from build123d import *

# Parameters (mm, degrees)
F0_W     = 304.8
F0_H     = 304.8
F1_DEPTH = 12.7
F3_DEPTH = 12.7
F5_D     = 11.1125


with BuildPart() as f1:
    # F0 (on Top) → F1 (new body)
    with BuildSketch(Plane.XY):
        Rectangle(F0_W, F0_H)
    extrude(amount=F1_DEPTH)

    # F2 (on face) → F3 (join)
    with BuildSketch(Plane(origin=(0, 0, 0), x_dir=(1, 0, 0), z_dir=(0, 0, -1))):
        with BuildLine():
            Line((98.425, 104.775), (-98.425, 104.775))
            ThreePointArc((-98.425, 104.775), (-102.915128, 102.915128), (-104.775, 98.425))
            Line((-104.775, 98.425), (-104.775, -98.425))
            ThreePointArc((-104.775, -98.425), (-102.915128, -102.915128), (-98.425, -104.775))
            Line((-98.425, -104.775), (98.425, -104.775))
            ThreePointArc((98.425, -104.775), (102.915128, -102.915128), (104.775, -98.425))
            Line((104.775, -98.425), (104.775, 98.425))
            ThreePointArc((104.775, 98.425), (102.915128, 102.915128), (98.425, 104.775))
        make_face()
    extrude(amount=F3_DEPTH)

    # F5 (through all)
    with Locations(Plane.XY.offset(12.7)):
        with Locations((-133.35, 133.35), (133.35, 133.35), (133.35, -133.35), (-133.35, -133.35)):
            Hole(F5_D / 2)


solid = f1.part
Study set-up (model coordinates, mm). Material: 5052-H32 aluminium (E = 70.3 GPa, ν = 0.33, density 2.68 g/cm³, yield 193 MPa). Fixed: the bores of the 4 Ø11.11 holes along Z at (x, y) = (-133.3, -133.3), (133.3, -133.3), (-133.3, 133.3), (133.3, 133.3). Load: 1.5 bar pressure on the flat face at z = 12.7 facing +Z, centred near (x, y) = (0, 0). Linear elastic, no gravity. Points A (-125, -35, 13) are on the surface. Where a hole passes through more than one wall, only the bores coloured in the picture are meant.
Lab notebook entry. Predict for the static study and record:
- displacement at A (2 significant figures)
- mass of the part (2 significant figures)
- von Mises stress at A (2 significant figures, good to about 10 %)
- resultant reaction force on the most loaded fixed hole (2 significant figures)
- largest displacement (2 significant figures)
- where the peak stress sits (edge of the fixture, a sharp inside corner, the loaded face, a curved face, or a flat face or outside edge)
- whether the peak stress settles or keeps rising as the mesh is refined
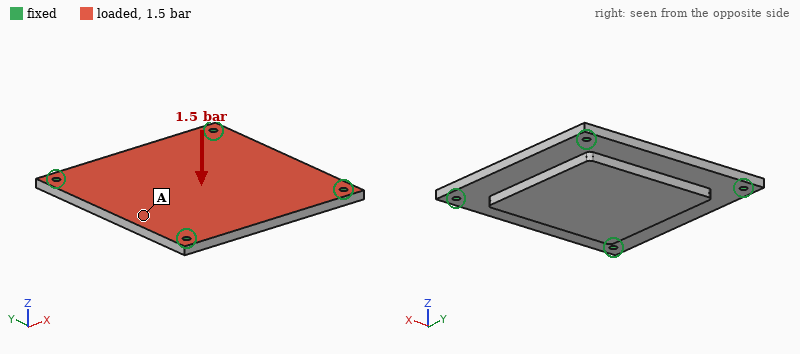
0.12 mm
4.6 kg
10 MPa
4.6 kN
0.16 mm
edge of the fixture
keeps rising
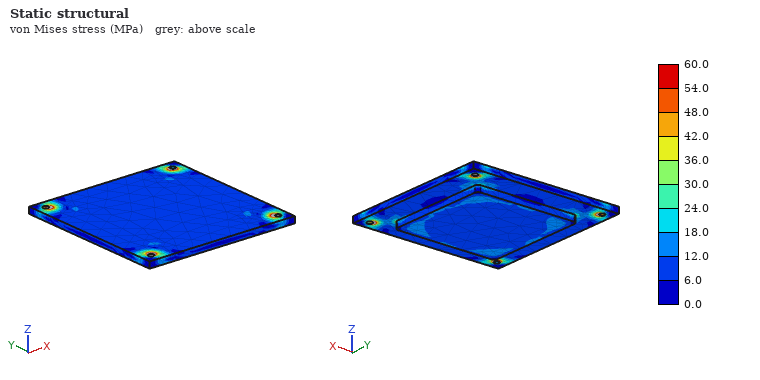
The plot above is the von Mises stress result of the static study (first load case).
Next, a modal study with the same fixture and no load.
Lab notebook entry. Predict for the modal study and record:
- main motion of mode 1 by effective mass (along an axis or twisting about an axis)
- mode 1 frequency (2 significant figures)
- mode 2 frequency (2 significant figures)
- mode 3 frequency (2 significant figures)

along Z
720 Hz
1200 Hz
1200 Hz
